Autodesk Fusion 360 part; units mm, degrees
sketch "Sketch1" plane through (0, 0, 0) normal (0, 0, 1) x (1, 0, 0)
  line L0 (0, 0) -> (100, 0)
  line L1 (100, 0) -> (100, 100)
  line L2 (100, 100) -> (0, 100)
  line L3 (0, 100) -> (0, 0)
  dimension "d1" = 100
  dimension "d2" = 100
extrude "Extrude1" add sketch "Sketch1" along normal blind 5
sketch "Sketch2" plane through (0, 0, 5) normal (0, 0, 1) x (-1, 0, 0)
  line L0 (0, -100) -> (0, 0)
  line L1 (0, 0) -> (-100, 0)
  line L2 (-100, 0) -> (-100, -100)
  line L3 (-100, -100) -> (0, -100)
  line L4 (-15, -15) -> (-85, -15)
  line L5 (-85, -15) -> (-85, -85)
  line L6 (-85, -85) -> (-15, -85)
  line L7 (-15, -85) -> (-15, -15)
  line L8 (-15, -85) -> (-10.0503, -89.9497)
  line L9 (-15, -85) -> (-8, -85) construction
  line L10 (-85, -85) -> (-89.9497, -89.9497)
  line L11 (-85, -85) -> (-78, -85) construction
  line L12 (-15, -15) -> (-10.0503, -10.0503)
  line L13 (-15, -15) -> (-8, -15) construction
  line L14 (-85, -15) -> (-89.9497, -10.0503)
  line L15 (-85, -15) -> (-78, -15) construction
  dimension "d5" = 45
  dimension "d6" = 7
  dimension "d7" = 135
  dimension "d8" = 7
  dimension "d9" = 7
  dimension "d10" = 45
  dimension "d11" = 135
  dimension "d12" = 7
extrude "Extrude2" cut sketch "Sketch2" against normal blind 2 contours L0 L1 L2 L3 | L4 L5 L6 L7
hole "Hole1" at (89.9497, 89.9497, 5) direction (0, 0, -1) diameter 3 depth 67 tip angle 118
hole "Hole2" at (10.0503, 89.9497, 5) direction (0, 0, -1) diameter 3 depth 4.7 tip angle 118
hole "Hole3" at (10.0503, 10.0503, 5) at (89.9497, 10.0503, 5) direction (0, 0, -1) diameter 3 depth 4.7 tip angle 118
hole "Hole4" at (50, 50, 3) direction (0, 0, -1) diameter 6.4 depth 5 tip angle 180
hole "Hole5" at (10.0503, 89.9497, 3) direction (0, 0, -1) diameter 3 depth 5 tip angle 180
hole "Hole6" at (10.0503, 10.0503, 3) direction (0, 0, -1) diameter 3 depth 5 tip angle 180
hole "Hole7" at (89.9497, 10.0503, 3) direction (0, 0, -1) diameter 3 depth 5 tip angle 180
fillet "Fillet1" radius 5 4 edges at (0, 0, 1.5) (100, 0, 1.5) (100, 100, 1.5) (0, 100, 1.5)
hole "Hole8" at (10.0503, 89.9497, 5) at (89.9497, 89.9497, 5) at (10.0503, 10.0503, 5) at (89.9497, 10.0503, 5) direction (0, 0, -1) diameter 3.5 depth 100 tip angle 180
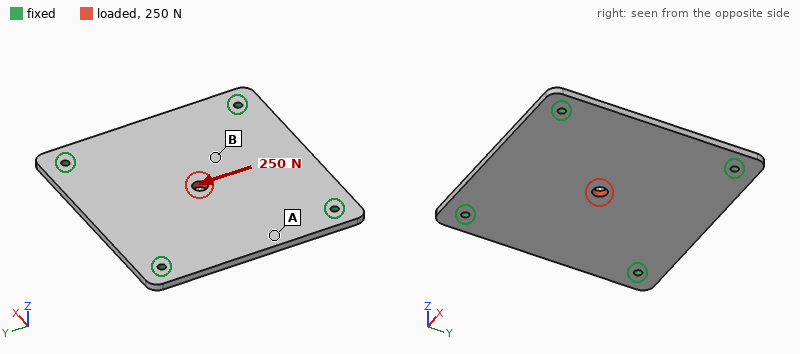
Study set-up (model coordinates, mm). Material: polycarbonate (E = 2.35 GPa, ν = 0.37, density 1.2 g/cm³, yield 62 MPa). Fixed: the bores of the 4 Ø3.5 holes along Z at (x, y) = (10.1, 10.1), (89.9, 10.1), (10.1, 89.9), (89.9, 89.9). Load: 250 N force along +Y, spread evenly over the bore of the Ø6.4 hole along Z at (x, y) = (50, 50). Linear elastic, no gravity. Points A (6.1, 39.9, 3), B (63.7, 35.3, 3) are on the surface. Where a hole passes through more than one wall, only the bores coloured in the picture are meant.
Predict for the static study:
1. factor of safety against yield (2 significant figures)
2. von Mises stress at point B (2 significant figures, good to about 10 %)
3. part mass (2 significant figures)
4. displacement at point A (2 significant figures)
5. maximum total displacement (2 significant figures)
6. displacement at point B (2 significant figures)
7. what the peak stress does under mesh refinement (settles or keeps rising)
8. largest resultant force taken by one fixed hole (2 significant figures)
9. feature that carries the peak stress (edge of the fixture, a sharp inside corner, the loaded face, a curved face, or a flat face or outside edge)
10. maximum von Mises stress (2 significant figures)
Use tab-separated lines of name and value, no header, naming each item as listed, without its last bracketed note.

factor of safety against yield	8.7
von Mises stress at point B	1.1 MPa
part mass	36 g
displacement at point A	7.8 µm
maximum total displacement	41 µm
displacement at point B	22 µm
what the peak stress does under mesh refinement	settles
largest resultant force taken by one fixed hole	70 N
feature that carries the peak stress	the loaded face
maximum von Mises stress	7.1 MPa
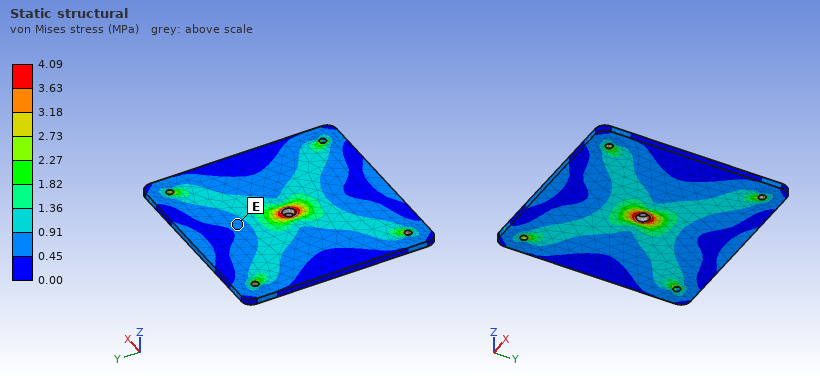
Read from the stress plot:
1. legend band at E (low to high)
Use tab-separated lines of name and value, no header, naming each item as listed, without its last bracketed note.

legend band at E	0.45 to 0.91 MPa
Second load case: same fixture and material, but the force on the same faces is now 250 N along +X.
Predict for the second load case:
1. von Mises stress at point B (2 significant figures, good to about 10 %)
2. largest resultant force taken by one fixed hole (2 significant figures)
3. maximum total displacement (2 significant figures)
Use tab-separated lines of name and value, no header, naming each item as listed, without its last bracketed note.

von Mises stress at point B	1.1 MPa
largest resultant force taken by one fixed hole	70 N
maximum total displacement	41 µm
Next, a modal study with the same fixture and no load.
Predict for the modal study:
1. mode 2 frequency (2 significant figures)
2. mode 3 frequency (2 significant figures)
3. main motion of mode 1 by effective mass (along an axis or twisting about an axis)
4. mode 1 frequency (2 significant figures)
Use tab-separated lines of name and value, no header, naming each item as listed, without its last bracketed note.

mode 2 frequency	730 Hz
mode 3 frequency	730 Hz
main motion of mode 1 by effective mass	along Z
mode 1 frequency	450 Hz
